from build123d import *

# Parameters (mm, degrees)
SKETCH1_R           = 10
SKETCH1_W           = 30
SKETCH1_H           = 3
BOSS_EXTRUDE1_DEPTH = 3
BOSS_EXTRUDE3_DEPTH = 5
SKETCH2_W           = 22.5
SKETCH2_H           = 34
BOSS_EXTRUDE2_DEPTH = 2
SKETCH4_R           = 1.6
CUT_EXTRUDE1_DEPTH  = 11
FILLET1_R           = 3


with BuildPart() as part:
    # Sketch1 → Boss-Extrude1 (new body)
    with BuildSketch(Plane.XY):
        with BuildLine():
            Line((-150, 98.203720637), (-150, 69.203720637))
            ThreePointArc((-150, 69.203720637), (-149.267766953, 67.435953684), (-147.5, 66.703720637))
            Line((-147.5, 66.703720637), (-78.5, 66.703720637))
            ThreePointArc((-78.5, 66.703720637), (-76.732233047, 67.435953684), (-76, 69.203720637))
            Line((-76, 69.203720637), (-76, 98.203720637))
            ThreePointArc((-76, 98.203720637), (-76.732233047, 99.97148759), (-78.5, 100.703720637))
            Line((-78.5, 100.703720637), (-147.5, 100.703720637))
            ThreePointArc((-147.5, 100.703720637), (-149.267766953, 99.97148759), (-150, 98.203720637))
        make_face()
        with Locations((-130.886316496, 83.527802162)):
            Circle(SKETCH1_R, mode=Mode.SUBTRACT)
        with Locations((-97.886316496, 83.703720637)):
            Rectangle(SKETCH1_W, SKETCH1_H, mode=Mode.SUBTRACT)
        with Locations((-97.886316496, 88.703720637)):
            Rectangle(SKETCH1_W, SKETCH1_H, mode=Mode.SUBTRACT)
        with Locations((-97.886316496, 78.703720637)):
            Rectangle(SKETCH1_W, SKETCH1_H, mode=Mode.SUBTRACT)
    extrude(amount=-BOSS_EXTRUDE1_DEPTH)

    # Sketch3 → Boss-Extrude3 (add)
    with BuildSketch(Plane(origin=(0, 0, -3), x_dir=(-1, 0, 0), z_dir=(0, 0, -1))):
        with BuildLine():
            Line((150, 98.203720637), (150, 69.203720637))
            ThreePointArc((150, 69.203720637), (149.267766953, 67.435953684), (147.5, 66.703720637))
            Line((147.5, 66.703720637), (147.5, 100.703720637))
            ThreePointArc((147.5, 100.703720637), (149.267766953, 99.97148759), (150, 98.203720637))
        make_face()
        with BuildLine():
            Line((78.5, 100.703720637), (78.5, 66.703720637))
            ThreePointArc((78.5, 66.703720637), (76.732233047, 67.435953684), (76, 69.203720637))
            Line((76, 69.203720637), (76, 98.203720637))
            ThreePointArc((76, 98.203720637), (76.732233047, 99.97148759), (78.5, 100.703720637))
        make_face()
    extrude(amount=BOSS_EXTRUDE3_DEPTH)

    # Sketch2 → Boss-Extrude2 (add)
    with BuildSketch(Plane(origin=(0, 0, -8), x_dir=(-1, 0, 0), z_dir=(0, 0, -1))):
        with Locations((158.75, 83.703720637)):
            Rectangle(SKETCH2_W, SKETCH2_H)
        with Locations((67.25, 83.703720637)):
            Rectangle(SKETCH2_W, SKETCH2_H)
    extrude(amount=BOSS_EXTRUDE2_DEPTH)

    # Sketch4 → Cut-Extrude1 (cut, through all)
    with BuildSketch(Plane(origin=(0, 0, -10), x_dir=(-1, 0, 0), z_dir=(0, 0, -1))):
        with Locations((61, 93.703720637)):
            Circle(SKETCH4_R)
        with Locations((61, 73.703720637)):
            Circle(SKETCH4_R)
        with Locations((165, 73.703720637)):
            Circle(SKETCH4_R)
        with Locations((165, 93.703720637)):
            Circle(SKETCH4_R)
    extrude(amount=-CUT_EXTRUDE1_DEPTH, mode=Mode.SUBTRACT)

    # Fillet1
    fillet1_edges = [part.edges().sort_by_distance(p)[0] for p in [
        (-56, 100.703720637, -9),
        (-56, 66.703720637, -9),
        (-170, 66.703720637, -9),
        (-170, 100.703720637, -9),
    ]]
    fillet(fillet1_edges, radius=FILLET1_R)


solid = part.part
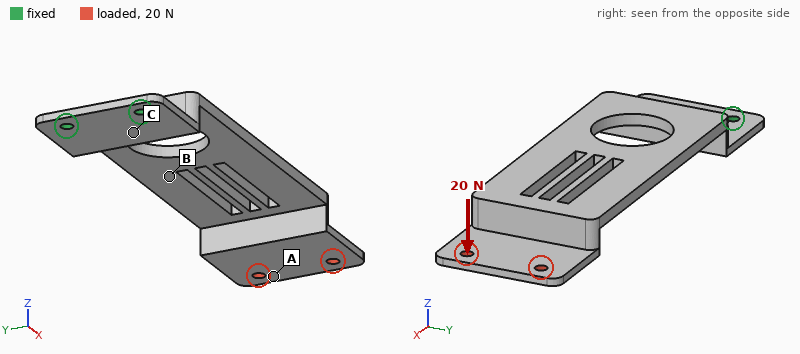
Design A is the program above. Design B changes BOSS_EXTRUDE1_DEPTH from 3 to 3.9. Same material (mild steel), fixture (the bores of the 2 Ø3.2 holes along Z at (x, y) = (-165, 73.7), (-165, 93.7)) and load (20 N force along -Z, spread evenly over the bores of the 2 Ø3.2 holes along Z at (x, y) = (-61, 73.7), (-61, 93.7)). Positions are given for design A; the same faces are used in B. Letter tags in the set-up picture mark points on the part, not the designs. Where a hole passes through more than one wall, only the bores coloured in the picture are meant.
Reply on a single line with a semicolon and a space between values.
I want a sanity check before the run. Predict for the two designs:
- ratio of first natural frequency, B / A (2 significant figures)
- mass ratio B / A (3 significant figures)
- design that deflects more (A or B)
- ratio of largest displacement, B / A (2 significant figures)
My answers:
1.0; 1.17; A; 0.77
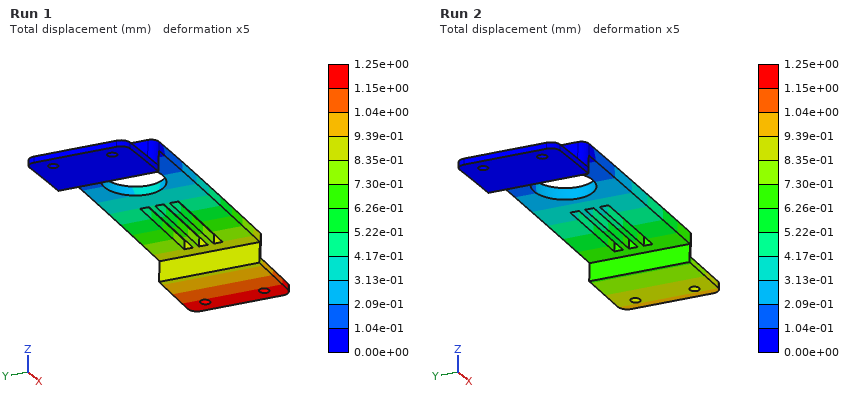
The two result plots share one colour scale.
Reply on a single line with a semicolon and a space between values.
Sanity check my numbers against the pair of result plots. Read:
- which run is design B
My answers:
Run 2
